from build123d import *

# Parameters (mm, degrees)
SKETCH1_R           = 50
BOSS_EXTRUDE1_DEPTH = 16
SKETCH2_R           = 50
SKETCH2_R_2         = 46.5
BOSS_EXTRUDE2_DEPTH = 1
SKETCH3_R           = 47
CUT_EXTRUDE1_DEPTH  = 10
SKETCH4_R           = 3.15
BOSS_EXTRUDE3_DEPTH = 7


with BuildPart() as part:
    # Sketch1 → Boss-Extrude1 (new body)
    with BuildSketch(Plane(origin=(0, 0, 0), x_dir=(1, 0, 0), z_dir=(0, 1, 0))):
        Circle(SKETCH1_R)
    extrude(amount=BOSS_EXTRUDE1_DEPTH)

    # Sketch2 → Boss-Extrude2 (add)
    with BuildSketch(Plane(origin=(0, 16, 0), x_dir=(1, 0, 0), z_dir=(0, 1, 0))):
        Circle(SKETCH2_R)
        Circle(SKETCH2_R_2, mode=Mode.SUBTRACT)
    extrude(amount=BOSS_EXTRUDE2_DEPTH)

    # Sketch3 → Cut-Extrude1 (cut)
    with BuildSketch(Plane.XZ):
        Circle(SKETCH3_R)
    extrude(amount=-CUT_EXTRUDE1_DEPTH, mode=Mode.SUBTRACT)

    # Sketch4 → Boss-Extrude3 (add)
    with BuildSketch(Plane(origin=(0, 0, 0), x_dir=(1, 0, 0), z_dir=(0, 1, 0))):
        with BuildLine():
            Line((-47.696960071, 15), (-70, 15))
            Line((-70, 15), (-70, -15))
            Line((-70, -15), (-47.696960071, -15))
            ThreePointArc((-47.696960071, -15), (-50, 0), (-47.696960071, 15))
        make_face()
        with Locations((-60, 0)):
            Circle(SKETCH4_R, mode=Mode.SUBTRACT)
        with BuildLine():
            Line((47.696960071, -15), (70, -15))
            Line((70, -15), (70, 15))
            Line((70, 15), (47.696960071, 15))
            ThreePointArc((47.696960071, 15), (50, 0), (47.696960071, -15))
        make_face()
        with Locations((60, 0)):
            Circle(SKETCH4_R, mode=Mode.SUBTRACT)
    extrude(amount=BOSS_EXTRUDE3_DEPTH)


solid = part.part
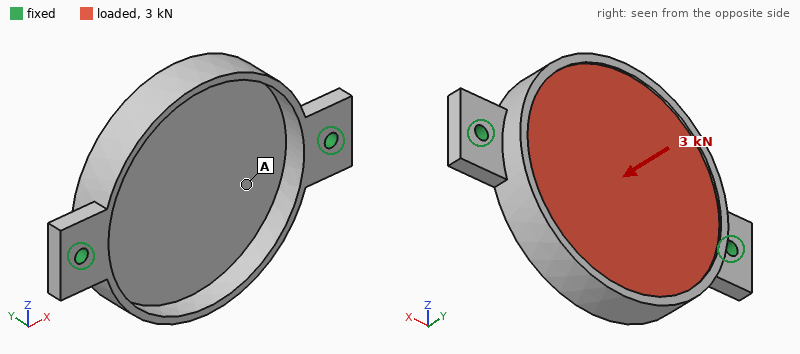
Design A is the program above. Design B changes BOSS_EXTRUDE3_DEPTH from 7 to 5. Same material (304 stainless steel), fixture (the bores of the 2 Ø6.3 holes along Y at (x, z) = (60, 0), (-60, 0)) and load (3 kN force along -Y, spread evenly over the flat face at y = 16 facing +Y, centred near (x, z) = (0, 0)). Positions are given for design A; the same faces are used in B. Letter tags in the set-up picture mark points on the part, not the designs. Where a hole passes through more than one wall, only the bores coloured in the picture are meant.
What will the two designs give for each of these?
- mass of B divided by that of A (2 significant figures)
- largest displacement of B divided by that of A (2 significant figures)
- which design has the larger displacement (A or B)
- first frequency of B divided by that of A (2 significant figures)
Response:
0.96
1.1
B
0.73
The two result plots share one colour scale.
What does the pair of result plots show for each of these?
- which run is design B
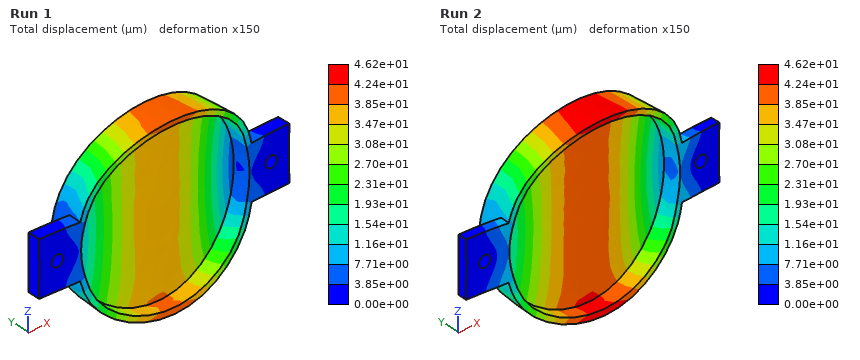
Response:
Run 2
